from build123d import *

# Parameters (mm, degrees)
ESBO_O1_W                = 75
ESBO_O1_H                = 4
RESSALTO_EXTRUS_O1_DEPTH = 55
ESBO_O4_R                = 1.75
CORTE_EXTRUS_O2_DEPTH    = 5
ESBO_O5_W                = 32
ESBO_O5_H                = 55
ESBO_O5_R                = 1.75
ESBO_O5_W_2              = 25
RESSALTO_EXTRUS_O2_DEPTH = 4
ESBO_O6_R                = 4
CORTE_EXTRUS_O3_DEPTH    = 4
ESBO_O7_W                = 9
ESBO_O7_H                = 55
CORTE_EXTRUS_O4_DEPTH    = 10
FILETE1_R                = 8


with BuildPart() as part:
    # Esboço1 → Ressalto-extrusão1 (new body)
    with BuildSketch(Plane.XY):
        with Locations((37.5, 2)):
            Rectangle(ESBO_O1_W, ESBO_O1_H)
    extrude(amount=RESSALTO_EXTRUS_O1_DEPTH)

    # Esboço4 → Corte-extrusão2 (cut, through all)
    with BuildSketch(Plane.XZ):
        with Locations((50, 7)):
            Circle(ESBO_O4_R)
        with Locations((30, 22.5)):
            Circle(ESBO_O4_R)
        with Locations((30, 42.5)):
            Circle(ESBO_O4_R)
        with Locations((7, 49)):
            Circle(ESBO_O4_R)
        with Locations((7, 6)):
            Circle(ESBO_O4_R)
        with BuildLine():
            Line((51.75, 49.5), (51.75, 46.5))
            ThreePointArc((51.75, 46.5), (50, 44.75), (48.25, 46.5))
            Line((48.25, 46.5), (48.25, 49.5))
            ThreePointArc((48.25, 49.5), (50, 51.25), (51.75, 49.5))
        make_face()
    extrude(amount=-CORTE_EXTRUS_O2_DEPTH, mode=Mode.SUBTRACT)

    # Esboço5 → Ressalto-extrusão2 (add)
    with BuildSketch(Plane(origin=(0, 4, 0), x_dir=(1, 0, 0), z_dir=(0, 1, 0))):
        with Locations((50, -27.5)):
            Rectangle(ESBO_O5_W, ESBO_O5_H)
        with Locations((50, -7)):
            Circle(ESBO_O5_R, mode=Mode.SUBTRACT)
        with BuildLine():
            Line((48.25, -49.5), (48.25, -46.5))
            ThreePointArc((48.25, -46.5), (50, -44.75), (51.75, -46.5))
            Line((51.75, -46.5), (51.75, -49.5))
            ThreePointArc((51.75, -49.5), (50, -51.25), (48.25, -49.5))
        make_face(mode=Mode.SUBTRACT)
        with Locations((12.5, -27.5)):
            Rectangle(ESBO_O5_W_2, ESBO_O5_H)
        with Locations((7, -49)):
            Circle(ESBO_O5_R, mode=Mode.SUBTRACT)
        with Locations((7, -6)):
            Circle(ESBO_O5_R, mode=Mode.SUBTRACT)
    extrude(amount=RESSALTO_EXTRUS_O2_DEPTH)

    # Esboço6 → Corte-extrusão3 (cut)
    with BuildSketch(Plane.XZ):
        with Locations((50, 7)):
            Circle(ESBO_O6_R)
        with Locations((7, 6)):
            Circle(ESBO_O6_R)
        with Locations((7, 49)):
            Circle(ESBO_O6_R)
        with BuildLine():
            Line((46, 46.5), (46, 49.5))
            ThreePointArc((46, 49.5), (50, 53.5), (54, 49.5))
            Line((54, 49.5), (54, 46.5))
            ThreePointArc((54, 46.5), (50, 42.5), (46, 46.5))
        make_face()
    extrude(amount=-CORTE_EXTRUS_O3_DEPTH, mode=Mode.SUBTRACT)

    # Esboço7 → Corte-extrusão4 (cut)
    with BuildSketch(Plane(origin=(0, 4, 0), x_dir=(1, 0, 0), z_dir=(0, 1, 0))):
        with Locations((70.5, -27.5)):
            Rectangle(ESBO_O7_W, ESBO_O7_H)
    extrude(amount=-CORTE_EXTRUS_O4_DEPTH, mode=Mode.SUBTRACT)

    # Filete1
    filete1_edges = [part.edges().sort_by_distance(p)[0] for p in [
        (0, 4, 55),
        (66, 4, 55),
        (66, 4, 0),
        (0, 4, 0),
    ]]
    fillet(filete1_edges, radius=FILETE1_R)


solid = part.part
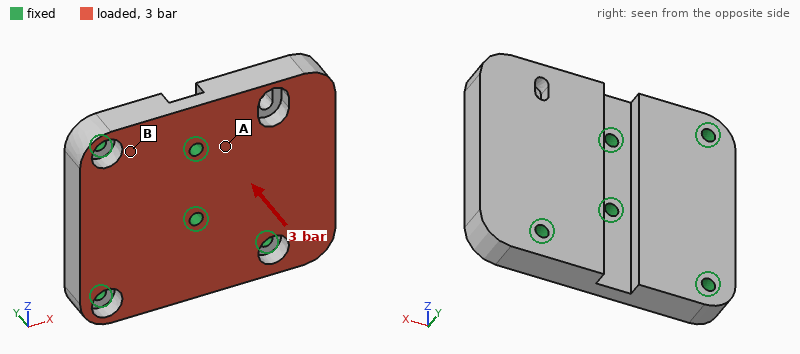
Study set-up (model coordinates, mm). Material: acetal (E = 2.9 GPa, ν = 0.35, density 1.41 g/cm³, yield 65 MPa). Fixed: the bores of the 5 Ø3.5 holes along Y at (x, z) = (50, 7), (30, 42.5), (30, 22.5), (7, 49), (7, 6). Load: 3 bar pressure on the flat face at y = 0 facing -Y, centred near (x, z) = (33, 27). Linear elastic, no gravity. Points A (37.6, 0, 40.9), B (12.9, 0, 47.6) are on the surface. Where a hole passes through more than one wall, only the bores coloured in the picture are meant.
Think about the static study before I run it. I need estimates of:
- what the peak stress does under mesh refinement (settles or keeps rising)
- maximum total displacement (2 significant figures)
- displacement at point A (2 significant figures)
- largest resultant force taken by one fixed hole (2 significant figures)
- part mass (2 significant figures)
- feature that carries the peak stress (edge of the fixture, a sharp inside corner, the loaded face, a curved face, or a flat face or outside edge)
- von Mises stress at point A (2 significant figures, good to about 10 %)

keeps rising
0.81 mm
0.13 mm
320 N
36 g
edge of the fixture
8.0 MPa
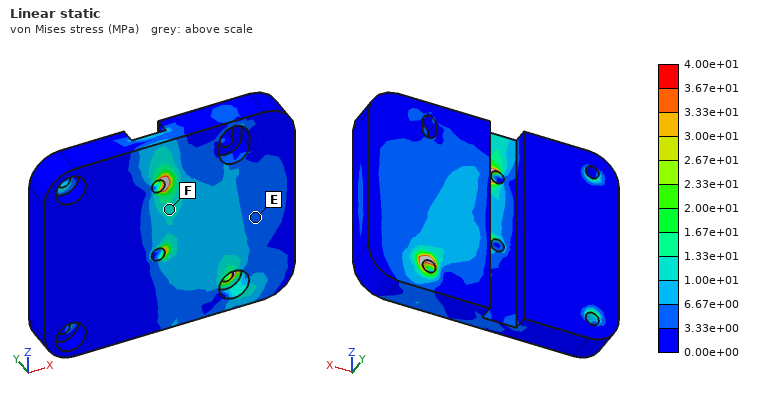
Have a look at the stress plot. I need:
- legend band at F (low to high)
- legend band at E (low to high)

1.00e+01 to 1.33e+01 MPa
3.33e+00 to 6.67e+00 MPa
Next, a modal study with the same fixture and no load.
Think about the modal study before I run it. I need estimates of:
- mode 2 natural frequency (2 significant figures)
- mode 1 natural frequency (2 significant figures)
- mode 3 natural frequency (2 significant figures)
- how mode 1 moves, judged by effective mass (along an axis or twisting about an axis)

3600 Hz
1200 Hz
4300 Hz
along Y
